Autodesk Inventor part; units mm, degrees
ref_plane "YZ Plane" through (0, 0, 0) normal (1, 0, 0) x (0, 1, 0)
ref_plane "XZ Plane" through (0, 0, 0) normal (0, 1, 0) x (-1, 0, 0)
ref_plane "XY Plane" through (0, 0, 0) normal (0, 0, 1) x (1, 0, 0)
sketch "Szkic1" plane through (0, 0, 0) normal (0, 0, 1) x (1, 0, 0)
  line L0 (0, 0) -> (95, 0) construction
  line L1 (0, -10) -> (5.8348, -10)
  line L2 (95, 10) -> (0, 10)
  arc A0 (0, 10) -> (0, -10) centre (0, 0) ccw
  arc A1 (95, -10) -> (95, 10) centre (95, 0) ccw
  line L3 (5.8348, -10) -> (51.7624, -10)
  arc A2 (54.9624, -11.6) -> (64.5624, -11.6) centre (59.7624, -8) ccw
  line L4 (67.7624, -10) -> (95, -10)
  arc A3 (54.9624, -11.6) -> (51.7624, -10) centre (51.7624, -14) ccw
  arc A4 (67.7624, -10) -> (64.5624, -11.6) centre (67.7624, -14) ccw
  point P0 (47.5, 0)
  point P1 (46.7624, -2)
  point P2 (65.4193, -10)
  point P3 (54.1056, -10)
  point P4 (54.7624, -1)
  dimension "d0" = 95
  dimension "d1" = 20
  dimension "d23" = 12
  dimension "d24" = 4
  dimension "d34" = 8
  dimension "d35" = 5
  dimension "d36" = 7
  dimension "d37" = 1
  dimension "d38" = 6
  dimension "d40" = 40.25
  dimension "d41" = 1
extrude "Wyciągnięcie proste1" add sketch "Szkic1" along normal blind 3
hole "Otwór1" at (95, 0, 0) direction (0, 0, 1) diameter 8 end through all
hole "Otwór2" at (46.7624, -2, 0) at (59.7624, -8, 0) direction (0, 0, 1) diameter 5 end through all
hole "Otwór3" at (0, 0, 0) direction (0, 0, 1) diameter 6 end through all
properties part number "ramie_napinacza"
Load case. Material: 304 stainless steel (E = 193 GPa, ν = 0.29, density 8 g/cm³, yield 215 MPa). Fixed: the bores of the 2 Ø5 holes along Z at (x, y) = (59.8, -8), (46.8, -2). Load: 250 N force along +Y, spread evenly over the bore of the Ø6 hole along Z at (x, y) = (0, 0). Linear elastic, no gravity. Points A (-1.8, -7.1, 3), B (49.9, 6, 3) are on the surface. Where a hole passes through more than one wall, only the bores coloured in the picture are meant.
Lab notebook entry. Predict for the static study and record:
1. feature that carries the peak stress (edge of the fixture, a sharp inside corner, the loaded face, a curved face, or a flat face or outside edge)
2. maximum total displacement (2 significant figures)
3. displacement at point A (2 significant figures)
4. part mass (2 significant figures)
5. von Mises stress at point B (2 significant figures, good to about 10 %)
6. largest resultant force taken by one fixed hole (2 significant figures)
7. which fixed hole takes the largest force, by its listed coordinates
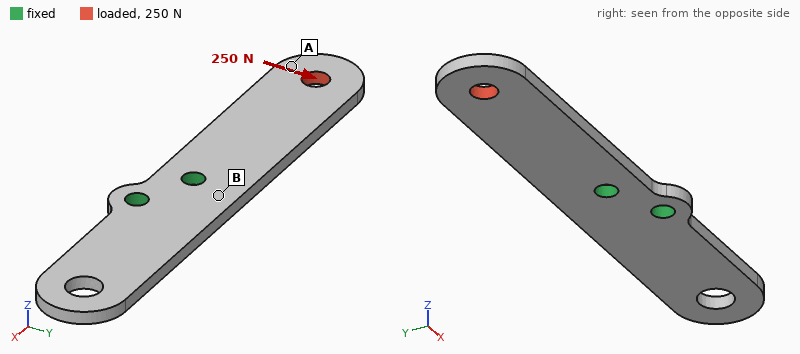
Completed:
edge of the fixture
46 µm
38 µm
51 g
26 MPa
710 N
(46.8, -2)
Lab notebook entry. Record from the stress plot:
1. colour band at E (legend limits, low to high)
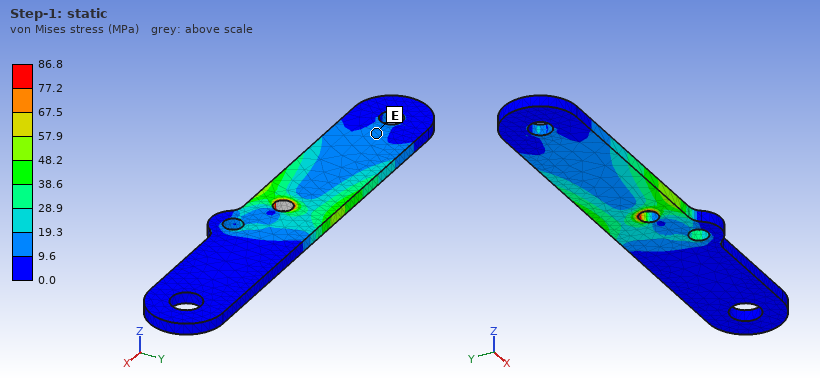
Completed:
9.6 to 19.3 MPa
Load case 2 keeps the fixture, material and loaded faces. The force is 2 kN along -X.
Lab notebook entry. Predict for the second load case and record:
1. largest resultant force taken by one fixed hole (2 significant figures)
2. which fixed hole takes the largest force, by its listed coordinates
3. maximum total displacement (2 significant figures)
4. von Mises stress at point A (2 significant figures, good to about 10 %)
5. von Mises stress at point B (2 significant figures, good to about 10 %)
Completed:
1.8 kN
(46.8, -2)
12 µm
17 MPa
19 MPa
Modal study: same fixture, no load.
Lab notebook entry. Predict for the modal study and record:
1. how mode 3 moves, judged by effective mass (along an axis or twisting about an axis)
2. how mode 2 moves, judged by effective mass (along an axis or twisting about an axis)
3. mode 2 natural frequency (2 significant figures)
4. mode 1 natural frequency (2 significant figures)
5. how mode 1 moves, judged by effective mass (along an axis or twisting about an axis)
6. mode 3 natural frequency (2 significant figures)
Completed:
along Y
along Z
1300 Hz
850 Hz
along Z
4100 Hz
